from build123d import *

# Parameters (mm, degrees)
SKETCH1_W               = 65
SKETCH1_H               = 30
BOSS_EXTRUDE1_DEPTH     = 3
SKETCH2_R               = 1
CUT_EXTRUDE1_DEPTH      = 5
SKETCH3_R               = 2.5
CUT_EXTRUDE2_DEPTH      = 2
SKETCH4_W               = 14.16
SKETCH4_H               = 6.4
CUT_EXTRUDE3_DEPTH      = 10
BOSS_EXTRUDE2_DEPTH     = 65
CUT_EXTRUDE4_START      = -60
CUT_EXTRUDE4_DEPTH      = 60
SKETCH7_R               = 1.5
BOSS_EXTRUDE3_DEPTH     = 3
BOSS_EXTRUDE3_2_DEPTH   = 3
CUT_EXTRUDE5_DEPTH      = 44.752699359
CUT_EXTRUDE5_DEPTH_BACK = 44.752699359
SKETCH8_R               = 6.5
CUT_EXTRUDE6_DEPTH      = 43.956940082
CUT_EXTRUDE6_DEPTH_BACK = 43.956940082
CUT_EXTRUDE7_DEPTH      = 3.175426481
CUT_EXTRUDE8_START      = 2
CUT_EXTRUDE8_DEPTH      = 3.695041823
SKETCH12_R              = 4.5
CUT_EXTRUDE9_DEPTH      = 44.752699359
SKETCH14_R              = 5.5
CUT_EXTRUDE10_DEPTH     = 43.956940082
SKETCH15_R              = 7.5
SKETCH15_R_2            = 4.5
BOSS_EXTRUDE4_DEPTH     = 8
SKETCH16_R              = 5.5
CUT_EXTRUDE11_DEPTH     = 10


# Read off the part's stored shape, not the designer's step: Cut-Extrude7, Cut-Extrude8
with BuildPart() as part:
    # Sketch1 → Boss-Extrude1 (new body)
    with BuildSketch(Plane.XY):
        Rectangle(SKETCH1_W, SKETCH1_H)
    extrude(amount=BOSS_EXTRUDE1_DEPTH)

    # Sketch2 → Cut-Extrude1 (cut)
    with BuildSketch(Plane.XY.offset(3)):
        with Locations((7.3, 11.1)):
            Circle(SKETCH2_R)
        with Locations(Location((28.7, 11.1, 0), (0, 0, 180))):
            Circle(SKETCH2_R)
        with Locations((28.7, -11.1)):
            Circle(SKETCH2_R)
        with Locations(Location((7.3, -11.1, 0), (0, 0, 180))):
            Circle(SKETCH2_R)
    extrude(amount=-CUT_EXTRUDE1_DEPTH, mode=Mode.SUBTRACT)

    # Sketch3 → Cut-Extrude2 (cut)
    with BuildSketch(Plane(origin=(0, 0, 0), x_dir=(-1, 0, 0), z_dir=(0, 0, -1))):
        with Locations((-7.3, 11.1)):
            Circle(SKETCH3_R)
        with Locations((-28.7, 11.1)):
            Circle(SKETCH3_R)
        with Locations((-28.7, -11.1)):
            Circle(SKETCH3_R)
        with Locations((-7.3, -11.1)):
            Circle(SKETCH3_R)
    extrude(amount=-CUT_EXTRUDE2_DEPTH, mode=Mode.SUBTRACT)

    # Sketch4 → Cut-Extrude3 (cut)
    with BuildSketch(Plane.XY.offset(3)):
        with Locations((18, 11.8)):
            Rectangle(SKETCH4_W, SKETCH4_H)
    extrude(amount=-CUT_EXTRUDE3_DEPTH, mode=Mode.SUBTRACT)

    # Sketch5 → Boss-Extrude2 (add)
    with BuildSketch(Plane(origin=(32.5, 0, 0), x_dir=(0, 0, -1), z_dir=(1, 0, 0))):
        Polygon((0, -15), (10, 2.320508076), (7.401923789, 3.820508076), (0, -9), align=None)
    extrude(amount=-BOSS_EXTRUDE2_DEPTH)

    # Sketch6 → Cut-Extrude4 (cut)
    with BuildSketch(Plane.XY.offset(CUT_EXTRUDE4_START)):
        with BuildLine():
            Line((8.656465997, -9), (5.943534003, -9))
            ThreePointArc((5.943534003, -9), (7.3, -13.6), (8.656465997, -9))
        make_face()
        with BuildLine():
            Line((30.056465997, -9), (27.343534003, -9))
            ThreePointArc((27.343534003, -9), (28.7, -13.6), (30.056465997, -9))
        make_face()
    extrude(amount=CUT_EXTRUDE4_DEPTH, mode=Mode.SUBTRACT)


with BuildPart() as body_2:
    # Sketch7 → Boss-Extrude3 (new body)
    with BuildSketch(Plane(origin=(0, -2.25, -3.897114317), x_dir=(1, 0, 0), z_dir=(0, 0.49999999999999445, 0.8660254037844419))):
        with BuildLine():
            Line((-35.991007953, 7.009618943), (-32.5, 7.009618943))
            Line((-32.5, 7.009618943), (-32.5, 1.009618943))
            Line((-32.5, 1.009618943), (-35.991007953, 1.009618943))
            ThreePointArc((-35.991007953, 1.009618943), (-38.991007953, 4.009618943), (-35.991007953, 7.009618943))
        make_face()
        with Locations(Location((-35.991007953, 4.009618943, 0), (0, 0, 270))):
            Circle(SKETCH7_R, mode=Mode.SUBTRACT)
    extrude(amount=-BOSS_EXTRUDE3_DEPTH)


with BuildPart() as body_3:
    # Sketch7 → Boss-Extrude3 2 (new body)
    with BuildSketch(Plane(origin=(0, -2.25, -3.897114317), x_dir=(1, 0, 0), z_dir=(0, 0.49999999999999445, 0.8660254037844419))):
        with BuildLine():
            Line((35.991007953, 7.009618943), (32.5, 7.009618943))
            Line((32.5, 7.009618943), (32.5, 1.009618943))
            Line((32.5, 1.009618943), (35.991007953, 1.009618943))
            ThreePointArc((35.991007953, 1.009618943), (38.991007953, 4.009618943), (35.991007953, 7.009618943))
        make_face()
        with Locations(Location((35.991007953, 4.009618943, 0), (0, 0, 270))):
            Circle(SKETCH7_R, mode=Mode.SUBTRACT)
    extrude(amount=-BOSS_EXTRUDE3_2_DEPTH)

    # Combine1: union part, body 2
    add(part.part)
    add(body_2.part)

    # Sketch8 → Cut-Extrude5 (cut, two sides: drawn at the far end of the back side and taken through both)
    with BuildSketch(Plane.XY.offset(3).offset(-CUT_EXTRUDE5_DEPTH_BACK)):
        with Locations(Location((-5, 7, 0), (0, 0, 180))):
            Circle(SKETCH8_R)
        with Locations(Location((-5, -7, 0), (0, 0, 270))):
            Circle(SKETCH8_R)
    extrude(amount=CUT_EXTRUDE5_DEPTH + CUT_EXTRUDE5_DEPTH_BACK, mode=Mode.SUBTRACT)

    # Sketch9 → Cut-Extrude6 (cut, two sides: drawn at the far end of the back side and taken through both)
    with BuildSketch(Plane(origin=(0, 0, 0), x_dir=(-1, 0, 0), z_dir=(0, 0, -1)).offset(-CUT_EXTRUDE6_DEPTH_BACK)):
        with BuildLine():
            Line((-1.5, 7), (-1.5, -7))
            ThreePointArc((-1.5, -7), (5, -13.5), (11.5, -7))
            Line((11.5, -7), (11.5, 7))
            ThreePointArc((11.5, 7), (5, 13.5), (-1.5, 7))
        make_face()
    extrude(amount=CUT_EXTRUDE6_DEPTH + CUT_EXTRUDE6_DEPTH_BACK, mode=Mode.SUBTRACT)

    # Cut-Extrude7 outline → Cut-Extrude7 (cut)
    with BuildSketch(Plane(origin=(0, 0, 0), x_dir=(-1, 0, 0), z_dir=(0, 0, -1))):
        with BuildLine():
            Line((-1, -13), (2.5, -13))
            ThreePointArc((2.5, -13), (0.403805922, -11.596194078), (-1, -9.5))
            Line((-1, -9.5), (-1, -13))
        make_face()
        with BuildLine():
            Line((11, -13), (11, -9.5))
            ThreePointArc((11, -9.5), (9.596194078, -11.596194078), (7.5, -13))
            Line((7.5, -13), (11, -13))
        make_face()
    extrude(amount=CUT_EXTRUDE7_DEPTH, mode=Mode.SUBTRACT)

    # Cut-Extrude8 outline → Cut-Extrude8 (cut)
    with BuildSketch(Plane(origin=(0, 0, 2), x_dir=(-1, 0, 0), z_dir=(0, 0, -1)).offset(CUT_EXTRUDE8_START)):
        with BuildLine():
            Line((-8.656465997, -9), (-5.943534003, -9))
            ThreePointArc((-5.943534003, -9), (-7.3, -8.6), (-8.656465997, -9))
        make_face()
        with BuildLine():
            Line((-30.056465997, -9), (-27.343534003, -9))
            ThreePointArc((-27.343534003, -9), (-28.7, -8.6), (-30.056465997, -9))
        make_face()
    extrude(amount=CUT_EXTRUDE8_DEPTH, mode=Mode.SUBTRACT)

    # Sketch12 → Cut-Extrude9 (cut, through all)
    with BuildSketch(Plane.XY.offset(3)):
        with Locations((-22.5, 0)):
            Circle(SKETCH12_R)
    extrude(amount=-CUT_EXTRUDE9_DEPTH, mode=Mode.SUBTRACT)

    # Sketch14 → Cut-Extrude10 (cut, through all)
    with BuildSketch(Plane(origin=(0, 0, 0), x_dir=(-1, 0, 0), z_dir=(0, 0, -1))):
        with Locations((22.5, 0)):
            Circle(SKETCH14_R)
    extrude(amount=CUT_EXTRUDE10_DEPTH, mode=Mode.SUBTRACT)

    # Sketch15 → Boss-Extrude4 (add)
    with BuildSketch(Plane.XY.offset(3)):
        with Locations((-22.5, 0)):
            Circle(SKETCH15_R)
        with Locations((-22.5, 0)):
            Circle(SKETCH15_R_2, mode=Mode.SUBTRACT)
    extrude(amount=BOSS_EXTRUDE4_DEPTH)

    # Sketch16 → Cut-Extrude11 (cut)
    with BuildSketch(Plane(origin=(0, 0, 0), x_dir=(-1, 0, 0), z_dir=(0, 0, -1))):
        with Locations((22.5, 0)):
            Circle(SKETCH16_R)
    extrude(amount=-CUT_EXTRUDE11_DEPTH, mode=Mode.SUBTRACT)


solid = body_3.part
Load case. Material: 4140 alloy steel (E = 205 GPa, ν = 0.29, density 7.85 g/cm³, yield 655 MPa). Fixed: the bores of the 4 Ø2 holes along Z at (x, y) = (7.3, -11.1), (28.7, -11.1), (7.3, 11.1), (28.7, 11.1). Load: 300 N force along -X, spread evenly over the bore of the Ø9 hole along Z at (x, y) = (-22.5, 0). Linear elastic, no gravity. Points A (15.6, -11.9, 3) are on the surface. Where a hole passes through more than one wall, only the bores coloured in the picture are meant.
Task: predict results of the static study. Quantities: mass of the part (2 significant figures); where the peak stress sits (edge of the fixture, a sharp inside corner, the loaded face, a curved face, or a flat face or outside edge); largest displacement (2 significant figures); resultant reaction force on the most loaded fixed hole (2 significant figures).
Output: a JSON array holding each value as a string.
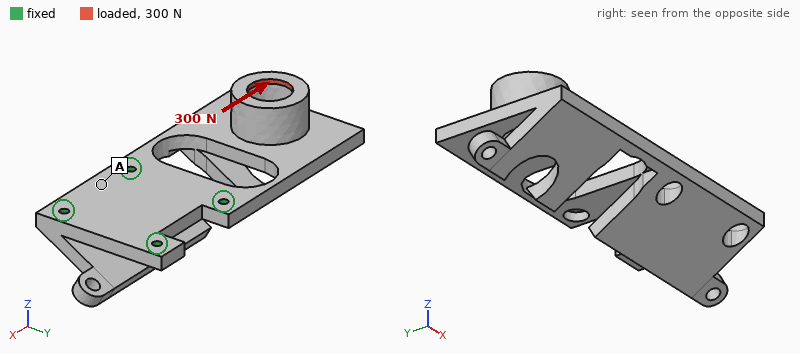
["58 g", "a curved face", "0.63 mm", "240 N"]
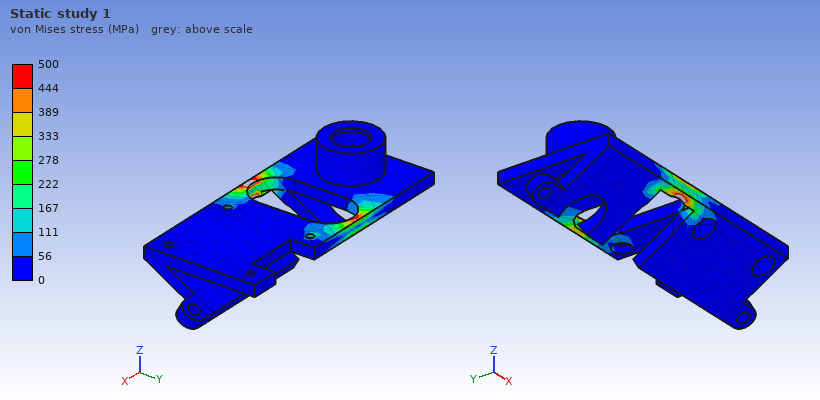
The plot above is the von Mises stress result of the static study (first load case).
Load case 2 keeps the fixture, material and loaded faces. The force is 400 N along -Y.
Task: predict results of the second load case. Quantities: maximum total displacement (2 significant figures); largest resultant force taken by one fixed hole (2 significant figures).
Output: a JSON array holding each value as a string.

["0.17 mm", "460 N"]
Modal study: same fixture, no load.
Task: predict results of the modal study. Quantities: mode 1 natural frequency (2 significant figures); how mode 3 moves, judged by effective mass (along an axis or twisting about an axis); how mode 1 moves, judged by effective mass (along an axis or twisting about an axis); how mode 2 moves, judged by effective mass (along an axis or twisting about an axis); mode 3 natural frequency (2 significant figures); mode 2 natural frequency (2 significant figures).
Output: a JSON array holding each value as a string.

["610 Hz", "twisting about X", "along Z", "along Y", "2800 Hz", "2600 Hz"]
